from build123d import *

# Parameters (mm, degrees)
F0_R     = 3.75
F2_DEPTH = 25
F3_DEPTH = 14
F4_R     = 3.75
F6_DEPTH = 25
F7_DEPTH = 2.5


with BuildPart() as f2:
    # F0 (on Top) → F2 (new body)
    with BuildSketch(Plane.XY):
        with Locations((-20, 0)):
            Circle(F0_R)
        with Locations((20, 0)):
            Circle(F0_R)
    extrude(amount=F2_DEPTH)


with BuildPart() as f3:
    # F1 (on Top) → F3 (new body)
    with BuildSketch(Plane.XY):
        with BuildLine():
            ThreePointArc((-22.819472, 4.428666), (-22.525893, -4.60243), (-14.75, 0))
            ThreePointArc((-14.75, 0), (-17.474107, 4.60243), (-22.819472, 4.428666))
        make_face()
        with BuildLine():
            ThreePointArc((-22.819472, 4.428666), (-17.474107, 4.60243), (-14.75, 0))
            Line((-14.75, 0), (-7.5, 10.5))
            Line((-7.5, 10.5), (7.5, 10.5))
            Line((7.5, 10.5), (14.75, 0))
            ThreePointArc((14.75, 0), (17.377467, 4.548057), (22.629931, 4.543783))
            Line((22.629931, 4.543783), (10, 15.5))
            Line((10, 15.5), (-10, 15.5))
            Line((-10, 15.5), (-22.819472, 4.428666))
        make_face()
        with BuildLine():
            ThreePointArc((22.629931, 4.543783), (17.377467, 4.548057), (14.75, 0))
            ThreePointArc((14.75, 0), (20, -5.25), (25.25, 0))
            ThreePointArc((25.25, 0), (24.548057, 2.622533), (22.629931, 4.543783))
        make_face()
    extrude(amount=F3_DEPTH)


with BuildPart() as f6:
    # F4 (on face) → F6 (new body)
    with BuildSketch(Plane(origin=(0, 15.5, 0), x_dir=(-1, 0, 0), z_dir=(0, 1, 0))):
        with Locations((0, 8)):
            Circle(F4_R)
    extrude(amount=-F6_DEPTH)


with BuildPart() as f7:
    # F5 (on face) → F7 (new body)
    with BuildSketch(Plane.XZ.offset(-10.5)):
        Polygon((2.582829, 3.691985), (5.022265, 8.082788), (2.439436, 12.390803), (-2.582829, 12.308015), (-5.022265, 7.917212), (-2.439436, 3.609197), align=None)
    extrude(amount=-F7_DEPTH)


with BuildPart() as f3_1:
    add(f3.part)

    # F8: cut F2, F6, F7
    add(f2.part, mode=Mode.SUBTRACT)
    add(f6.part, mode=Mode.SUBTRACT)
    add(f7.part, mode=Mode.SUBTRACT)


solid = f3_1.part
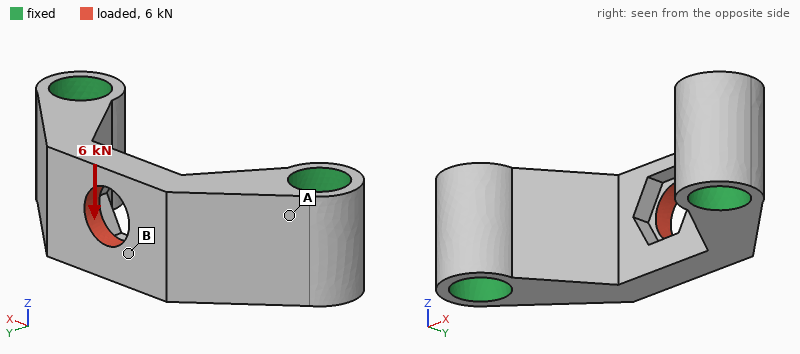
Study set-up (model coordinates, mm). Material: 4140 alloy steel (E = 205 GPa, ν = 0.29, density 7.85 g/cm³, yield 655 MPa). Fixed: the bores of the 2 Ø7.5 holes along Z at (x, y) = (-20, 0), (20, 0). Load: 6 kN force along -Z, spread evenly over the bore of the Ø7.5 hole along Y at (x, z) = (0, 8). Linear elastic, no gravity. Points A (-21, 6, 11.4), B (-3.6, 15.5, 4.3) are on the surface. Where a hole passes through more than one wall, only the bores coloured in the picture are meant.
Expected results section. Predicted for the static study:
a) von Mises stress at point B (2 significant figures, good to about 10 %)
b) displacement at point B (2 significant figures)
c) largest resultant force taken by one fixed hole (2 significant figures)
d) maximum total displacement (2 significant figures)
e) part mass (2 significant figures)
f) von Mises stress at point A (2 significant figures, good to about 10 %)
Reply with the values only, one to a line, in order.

130 MPa
24 µm
3.0 kN
32 µm
36 g
43 MPa
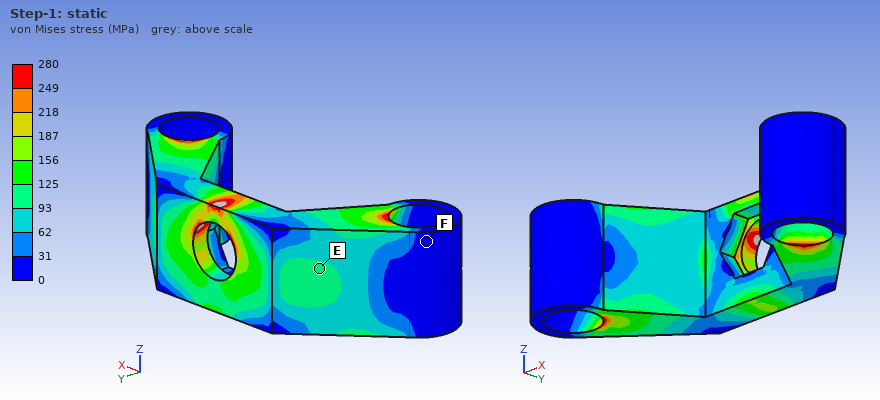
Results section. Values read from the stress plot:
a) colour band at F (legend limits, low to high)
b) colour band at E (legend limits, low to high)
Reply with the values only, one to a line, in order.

0 to 31 MPa
93 to 125 MPa
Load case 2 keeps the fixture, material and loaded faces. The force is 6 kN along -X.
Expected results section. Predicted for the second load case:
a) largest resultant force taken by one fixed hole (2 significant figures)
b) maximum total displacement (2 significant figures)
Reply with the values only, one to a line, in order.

3.2 kN
13 µm
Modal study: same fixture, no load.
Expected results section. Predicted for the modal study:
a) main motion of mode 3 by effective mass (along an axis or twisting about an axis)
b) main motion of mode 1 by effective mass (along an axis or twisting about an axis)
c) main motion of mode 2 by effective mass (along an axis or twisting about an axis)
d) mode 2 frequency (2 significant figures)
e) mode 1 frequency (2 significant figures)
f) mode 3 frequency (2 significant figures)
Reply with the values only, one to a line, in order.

along Y
along Z
along X
29 kHz
27 kHz
36 kHz
